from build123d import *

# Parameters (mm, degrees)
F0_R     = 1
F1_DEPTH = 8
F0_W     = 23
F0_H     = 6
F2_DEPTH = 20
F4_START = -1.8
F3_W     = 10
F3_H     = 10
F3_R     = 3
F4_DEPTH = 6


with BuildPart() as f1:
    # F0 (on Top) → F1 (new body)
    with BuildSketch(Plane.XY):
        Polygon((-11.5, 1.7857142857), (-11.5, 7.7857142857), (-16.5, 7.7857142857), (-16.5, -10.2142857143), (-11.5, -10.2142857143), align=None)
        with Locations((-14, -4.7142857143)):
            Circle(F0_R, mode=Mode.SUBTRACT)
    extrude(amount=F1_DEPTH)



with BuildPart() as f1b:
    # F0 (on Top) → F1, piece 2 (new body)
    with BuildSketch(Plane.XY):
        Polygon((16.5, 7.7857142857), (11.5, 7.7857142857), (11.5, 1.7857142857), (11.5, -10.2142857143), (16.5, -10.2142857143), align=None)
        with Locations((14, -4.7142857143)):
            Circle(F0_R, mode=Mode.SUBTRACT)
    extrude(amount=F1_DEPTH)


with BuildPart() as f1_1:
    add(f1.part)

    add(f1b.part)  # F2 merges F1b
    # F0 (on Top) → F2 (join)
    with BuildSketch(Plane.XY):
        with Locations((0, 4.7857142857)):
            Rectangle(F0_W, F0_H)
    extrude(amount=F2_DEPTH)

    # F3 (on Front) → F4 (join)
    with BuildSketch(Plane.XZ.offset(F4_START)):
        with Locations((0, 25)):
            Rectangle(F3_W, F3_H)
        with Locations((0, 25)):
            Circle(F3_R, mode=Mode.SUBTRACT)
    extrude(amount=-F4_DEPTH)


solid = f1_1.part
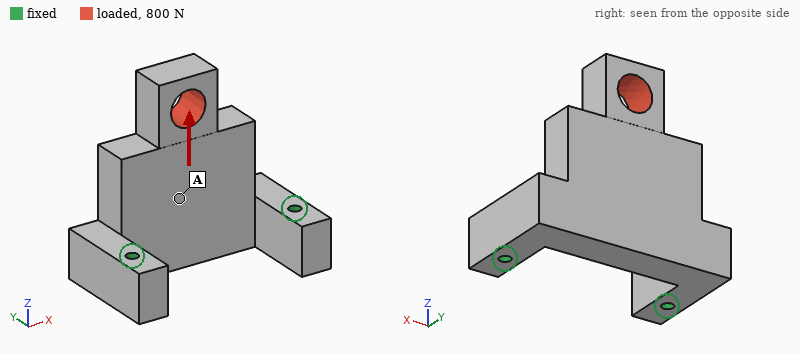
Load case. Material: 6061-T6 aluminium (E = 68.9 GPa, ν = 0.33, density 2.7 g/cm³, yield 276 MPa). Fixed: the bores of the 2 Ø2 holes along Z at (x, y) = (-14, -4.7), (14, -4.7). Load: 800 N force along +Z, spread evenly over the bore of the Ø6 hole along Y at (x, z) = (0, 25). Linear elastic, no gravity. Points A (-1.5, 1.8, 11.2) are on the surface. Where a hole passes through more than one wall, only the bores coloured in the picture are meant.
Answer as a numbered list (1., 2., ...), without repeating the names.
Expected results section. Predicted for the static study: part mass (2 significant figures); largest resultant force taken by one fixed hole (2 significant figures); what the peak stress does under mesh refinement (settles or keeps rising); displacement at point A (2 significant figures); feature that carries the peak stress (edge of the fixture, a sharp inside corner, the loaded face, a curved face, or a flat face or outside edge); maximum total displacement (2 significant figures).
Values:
1. 12 g
2. 400 N
3. keeps rising
4. 15 µm
5. edge of the fixture
6. 42 µm
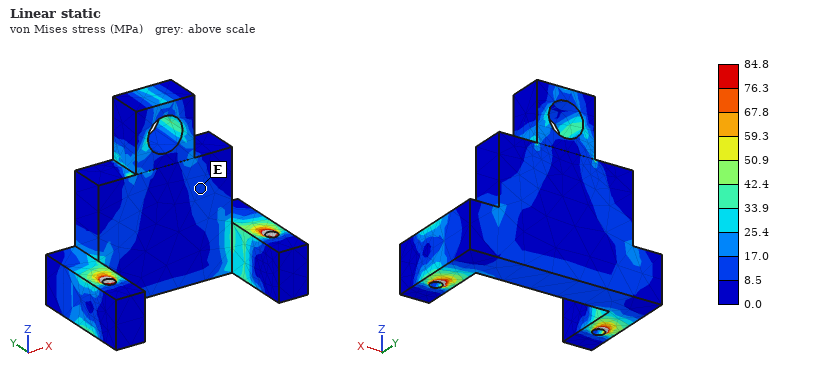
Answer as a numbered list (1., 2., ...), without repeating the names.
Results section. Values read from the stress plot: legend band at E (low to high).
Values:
1. 8.5 to 17.0 MPa
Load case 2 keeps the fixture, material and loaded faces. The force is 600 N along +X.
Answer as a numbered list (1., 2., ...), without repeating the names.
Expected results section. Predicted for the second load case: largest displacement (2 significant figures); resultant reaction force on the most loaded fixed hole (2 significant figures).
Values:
1. 50 µm
2. 540 N
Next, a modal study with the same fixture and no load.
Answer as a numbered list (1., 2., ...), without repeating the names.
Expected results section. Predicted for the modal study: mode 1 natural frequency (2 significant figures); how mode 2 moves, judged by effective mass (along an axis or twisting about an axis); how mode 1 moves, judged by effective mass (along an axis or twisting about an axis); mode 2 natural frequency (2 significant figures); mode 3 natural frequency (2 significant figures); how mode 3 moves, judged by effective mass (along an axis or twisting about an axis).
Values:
1. 5800 Hz
2. along X
3. along Y
4. 12 kHz
5. 14 kHz
6. along Z
